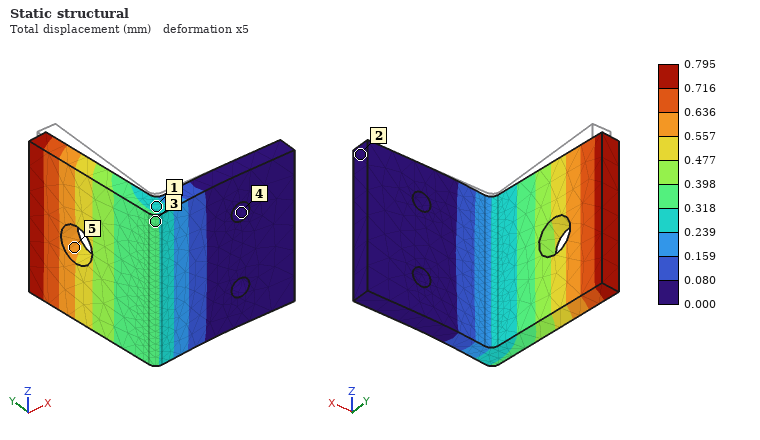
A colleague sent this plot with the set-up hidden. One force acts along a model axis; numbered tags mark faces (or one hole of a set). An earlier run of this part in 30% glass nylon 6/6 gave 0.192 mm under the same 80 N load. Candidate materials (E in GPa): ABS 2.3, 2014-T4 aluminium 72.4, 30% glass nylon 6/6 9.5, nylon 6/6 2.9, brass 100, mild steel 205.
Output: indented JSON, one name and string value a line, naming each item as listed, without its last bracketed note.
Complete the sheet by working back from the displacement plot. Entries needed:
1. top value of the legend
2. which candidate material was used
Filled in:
{
  "top value of the legend": "0.795 mm",
  "which candidate material was used": "ABS"
}
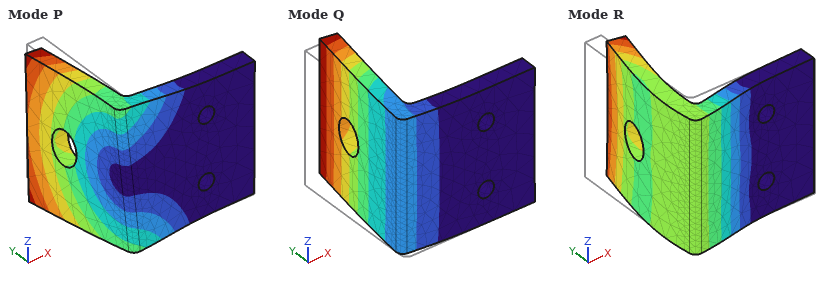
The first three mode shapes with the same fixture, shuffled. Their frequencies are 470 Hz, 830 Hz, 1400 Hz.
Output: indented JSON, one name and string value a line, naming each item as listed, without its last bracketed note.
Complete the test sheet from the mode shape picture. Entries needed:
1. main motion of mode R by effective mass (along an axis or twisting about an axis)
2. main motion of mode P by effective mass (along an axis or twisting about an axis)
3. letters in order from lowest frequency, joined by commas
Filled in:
{
  "main motion of mode R by effective mass": "along Y",
  "main motion of mode P by effective mass": "along Z",
  "letters in order from lowest frequency, joined by commas": "Q, P, R"
}
